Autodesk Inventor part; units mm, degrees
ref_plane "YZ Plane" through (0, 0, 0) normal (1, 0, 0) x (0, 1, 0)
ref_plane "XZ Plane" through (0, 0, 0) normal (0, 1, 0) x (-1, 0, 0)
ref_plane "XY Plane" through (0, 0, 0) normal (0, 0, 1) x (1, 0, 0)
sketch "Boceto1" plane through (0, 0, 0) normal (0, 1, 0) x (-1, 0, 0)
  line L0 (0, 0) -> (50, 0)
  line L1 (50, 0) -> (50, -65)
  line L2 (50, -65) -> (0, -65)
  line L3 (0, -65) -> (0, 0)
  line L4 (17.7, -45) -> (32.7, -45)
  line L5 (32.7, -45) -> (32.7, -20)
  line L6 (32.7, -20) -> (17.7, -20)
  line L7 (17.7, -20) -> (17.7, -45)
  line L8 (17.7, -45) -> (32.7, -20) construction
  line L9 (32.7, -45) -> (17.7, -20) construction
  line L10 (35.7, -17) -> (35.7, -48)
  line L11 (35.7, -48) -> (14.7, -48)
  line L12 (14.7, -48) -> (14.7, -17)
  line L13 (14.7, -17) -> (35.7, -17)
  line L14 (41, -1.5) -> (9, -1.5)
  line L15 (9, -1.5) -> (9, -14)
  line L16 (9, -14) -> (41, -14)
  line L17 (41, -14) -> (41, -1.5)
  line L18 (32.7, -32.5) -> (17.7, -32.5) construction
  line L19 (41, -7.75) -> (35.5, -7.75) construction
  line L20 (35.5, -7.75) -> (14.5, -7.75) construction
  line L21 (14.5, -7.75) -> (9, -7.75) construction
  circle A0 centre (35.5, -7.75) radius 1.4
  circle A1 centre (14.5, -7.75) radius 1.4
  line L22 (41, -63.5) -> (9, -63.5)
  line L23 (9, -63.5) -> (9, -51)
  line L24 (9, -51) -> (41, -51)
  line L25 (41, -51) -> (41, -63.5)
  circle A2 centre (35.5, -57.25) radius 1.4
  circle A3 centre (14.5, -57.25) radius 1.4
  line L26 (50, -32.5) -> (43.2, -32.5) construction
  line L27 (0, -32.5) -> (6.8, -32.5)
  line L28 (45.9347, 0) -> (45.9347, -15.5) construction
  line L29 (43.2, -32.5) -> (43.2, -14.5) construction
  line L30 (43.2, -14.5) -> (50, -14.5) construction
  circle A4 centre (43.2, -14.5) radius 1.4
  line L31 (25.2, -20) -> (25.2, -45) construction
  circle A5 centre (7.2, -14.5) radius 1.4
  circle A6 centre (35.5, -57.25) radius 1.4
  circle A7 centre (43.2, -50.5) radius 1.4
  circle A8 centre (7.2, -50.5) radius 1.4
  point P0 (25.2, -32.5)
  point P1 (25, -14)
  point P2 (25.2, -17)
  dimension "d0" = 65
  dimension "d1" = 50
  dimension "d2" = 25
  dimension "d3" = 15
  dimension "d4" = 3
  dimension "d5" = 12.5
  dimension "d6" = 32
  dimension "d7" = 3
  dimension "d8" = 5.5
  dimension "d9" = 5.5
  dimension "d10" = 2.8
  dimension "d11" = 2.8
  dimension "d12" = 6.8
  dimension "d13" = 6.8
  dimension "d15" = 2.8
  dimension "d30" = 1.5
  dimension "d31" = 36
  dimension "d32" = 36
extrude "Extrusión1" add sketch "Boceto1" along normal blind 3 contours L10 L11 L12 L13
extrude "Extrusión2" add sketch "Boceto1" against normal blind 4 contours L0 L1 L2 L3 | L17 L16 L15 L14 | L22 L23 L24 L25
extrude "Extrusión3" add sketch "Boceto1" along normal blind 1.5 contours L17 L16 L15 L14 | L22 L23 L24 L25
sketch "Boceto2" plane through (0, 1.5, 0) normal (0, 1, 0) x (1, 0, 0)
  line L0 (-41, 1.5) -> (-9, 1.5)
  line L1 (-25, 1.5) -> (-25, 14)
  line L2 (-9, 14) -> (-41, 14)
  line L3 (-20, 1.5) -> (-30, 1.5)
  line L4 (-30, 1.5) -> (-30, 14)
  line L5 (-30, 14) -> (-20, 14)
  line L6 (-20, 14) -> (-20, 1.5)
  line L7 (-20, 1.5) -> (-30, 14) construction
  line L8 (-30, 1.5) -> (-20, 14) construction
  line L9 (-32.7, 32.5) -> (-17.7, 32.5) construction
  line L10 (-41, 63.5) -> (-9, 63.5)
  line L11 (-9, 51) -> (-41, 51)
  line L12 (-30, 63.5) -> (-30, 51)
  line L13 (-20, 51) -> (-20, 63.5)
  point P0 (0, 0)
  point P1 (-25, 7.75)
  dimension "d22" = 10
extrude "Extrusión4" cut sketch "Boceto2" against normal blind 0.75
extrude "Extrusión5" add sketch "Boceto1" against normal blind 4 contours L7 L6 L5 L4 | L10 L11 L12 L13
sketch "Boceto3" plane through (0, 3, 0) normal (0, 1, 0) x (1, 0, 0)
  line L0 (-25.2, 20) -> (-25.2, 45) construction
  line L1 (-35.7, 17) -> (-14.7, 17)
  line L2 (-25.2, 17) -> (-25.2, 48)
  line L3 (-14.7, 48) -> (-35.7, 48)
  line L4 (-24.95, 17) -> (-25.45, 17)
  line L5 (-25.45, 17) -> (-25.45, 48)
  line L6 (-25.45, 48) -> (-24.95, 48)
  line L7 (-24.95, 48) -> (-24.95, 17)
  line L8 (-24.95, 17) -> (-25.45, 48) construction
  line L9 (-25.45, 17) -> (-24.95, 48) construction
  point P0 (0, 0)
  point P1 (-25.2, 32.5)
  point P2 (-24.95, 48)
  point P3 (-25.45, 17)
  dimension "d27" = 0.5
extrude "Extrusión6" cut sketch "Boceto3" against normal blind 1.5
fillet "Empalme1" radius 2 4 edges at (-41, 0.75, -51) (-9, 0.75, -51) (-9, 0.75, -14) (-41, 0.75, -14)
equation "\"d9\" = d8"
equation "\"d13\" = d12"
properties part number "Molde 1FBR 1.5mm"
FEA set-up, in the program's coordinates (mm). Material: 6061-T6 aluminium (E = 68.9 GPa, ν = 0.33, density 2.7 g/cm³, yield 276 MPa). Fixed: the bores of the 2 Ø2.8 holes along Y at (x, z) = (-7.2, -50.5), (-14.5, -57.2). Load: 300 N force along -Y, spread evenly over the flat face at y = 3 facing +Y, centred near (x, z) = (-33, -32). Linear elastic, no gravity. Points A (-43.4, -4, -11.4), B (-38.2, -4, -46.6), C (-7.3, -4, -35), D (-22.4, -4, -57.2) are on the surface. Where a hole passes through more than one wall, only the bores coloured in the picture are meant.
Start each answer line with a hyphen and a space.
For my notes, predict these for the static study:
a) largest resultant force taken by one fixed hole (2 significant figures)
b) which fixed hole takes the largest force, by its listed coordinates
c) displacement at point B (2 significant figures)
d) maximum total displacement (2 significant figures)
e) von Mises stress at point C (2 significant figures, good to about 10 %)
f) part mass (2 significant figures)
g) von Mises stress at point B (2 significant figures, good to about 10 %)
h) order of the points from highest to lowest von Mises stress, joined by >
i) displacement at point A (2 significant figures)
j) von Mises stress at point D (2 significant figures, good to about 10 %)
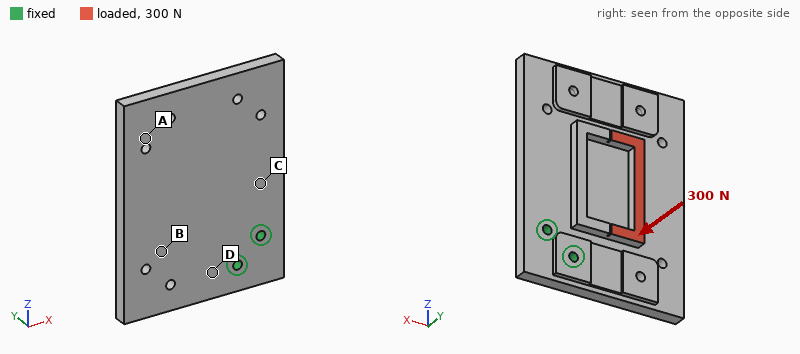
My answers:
- 240 N
- (-14.5, -57.2)
- 0.10 mm
- 0.42 mm
- 28 MPa
- 39 g
- 15 MPa
- D > C > B > A
- 0.33 mm
- 54 MPa
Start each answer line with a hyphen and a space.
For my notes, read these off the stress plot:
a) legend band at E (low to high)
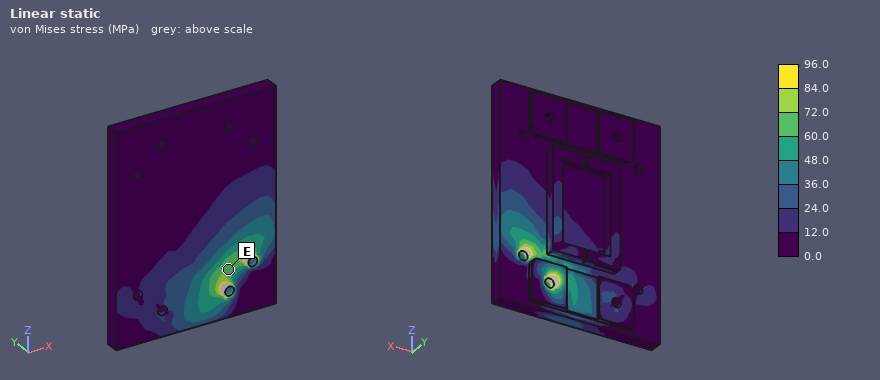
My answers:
- 60.0 to 72.0 MPa
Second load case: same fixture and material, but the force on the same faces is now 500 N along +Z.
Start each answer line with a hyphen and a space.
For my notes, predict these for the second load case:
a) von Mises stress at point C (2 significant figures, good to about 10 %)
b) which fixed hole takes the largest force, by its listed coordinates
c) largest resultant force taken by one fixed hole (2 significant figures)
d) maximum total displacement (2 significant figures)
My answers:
- 11 MPa
- (-14.5, -57.2)
- 1.1 kN
- 0.13 mm
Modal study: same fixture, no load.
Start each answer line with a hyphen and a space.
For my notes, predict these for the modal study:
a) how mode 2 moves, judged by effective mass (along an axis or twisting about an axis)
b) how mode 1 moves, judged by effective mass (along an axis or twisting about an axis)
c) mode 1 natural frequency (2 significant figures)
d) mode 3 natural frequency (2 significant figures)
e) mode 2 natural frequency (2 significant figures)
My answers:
- twisting about Z
- along Y
- 970 Hz
- 3300 Hz
- 2300 Hz
